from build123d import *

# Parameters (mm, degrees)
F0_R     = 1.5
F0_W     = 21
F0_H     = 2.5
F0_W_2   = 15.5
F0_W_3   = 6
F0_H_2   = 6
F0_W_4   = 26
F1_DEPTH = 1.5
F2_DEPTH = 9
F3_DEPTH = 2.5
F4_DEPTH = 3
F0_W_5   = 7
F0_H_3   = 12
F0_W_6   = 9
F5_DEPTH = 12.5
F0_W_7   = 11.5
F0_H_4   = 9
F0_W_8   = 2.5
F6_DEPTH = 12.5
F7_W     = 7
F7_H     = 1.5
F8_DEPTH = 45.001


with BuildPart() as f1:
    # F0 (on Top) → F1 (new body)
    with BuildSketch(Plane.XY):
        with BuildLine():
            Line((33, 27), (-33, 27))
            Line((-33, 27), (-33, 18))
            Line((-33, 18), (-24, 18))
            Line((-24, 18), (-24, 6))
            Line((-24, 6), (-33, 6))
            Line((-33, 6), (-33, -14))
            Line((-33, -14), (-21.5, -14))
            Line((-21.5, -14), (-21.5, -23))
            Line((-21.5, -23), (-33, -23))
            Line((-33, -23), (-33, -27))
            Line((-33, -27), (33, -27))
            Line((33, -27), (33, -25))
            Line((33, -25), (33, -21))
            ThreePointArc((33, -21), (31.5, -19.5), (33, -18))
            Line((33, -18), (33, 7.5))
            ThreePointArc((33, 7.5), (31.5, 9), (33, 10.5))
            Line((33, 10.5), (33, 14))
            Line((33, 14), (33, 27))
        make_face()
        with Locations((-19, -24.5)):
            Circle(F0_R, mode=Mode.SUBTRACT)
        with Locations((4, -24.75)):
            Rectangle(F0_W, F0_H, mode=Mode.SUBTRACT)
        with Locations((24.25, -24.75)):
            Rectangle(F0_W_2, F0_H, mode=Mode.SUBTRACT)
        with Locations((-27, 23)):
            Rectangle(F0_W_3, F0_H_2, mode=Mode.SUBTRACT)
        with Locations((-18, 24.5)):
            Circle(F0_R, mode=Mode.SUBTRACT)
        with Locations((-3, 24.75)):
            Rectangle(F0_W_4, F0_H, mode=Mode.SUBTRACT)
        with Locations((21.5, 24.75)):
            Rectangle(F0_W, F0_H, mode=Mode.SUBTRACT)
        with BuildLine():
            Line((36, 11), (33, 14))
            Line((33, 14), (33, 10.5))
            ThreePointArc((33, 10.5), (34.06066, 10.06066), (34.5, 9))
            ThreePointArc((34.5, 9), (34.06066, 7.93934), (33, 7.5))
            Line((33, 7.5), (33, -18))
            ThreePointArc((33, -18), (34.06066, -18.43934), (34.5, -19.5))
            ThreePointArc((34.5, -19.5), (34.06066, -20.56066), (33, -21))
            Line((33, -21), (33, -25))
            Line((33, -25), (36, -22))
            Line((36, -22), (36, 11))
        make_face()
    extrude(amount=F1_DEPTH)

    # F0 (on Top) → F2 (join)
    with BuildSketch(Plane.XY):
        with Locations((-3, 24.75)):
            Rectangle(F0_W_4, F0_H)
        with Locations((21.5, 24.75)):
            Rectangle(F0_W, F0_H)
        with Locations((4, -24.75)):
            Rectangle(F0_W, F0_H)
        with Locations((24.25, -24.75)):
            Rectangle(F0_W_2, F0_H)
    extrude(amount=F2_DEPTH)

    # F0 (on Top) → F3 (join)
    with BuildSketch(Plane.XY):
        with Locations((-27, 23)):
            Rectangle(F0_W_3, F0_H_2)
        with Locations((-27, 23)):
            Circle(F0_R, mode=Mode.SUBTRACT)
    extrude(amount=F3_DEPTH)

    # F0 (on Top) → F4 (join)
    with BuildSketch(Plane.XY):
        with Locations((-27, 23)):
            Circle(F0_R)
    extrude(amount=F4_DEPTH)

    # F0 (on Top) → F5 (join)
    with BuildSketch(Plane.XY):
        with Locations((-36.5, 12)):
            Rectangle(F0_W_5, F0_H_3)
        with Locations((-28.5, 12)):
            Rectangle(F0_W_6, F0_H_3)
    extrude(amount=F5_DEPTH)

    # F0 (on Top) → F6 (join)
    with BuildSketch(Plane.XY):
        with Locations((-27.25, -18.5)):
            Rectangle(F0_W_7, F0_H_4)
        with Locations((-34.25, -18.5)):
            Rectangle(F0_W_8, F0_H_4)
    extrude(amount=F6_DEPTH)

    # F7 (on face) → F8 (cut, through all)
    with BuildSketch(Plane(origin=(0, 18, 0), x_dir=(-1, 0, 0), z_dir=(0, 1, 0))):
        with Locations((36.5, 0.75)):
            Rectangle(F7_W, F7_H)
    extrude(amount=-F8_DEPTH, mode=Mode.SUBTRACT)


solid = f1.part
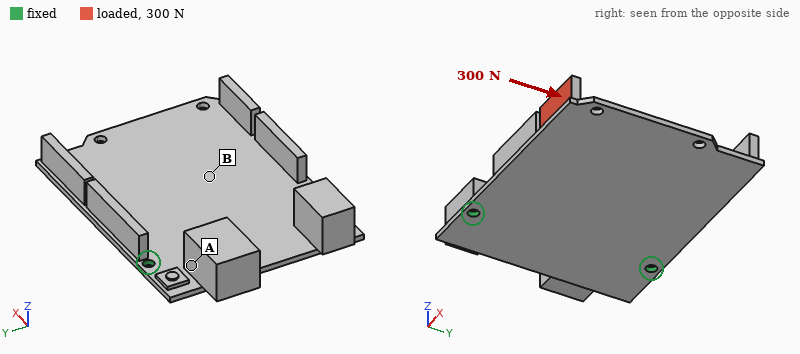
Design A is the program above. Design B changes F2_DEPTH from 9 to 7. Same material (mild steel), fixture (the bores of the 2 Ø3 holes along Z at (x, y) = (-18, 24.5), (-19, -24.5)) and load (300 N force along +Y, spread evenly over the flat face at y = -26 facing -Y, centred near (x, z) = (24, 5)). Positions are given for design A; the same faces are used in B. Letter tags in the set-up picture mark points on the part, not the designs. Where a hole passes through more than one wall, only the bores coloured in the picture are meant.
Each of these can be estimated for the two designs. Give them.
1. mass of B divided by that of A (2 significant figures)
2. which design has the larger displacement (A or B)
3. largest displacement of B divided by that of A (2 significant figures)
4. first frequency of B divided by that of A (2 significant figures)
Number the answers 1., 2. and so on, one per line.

1. 0.96
2. A
3. 0.74
4. 1.0
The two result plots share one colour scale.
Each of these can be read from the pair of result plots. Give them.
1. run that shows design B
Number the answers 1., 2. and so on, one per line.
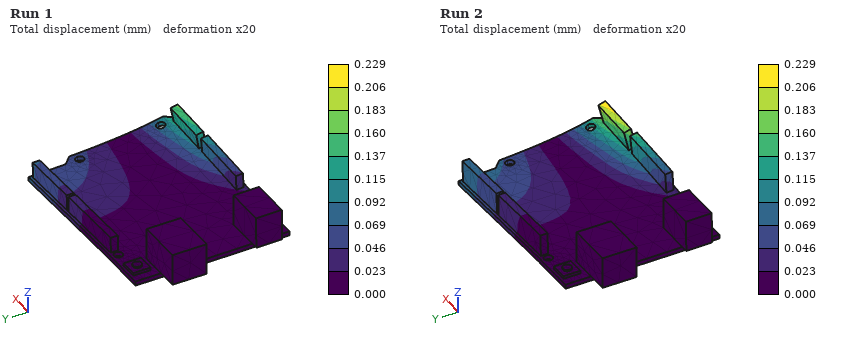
1. Run 1
